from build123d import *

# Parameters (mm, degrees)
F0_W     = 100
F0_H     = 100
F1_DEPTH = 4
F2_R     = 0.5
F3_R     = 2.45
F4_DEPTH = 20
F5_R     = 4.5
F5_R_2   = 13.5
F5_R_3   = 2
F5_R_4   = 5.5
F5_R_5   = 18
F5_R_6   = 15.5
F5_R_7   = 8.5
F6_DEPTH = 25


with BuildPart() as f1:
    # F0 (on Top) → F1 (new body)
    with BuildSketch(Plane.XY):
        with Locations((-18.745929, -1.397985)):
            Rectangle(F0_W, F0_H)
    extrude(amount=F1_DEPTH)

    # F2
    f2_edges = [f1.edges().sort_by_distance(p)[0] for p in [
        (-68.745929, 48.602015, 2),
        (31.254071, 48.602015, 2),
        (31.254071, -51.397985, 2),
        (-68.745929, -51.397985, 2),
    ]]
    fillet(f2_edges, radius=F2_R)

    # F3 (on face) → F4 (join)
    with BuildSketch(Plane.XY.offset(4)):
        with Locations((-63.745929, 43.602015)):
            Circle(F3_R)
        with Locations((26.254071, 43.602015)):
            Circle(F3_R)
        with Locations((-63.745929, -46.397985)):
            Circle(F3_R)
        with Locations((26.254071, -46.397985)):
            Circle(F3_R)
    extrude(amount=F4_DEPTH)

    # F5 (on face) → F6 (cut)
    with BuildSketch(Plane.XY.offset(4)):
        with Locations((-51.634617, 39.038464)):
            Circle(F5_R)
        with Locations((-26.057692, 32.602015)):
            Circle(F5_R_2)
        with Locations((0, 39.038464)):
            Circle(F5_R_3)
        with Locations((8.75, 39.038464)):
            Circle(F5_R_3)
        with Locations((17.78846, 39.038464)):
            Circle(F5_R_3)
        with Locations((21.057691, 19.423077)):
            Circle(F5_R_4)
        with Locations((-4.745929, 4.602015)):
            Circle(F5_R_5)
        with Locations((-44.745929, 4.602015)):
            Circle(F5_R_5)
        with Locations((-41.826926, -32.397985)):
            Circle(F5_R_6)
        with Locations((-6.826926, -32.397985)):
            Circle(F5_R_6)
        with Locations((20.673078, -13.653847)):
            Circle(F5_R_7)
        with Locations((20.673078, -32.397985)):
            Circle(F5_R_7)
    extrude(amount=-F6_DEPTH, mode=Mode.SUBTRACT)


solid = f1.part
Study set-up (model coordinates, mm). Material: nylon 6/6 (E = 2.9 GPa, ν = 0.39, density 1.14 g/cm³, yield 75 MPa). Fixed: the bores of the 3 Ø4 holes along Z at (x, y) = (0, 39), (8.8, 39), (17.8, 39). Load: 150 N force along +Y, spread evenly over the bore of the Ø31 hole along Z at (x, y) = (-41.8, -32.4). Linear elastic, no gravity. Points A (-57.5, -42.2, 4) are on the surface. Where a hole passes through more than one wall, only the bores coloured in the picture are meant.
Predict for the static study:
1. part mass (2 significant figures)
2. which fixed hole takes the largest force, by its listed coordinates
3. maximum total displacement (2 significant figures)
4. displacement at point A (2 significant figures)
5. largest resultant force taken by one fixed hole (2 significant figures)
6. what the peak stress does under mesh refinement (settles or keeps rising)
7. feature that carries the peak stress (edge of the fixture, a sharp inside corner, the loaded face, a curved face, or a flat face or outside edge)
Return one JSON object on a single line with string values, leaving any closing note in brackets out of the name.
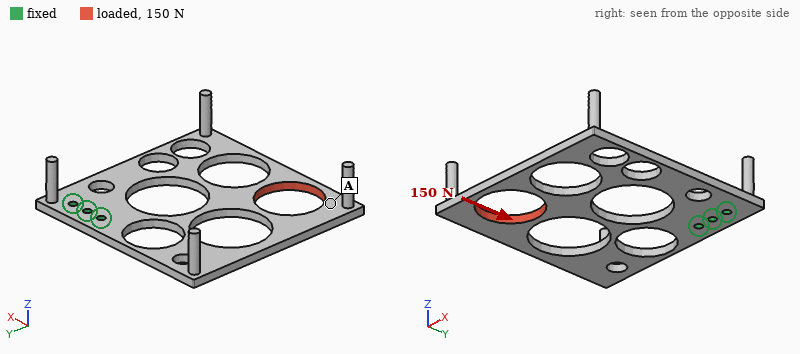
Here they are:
{"part mass": "26 g", "which fixed hole takes the largest force, by its listed coordinates": "(0, 39)", "maximum total displacement": "1.4 mm", "displacement at point A": "1.3 mm", "largest resultant force taken by one fixed hole": "410 N", "what the peak stress does under mesh refinement": "keeps rising", "feature that carries the peak stress": "a sharp inside corner"}
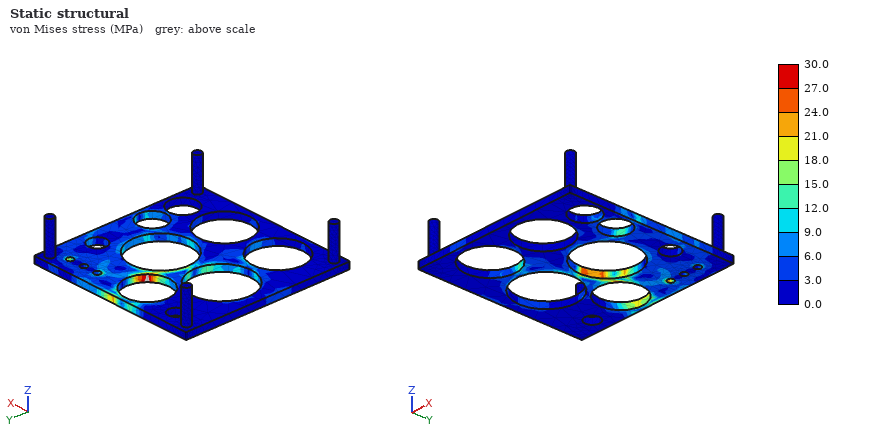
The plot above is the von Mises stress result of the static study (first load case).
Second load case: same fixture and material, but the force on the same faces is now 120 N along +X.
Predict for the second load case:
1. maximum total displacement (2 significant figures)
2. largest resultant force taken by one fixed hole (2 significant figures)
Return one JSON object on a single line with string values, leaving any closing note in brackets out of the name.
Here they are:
{"maximum total displacement": "1.5 mm", "largest resultant force taken by one fixed hole": "410 N"}
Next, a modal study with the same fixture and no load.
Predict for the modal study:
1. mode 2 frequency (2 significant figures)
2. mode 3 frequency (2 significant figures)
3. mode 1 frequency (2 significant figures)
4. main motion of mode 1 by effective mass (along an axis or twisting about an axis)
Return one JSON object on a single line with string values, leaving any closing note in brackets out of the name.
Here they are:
{"mode 2 frequency": "130 Hz", "mode 3 frequency": "230 Hz", "mode 1 frequency": "70 Hz", "main motion of mode 1 by effective mass": "along Z"}
